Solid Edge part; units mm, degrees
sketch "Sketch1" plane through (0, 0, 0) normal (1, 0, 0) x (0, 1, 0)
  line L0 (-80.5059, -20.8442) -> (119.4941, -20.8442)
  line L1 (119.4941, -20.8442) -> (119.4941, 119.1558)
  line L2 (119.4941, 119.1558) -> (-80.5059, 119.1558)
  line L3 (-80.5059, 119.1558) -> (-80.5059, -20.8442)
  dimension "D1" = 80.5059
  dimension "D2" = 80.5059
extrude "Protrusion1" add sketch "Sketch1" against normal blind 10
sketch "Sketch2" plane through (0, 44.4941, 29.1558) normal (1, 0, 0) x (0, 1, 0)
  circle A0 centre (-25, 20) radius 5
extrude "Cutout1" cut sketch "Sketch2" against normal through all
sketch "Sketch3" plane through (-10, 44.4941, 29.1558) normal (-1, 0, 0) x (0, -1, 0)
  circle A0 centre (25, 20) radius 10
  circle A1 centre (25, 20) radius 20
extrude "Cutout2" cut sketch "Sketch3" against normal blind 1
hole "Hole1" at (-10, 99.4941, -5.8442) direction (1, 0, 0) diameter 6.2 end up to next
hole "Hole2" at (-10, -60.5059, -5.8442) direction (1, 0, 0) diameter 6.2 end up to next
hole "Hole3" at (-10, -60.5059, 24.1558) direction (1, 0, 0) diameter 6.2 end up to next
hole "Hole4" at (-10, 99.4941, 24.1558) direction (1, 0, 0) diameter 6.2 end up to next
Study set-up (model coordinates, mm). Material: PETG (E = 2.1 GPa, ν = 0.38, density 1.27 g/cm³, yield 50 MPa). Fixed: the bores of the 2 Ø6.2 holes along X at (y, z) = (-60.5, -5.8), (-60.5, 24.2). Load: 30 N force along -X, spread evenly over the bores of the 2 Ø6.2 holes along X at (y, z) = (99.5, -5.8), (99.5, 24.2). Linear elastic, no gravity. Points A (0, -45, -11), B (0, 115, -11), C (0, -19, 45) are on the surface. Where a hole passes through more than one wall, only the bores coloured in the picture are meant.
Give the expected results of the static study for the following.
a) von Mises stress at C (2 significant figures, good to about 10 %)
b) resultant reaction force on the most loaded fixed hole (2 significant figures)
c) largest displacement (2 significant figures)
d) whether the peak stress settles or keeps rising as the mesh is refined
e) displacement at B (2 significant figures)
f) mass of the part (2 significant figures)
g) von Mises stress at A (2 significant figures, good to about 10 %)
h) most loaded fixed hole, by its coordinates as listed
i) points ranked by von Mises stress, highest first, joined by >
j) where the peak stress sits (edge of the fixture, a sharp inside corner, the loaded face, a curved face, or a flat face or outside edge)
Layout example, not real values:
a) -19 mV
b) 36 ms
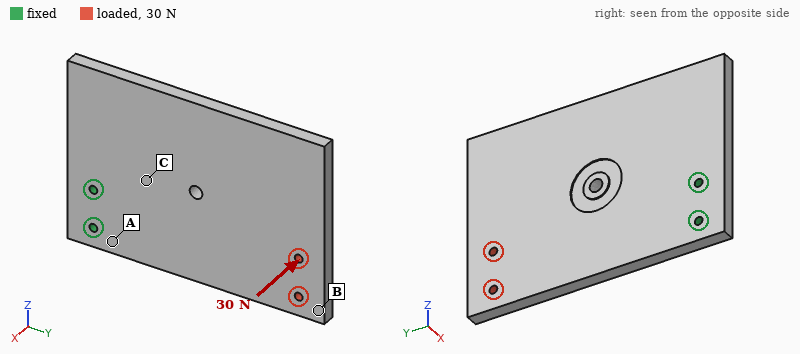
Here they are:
a) 1.5 MPa
b) 17 N
c) 2.9 mm
d) keeps rising
e) 2.8 mm
f) 350 g
g) 2.9 MPa
h) (-60.5, 24.2)
i) A > C > B
j) edge of the fixture
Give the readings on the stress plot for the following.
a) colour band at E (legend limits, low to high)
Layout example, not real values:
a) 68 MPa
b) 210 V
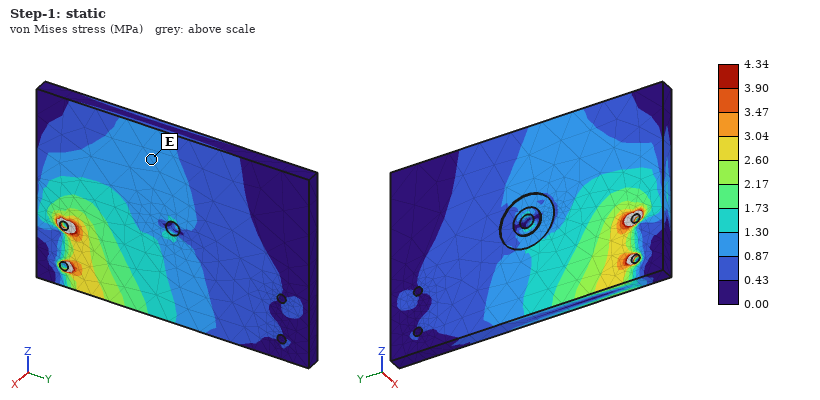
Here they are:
a) 0.87 to 1.30 MPa
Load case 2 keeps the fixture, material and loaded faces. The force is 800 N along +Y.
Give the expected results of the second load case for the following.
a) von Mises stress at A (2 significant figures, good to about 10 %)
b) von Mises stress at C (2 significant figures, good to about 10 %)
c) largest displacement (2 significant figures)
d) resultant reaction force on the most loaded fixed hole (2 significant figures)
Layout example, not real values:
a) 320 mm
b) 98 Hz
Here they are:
a) 1.5 MPa
b) 0.56 MPa
c) 0.14 mm
d) 400 N
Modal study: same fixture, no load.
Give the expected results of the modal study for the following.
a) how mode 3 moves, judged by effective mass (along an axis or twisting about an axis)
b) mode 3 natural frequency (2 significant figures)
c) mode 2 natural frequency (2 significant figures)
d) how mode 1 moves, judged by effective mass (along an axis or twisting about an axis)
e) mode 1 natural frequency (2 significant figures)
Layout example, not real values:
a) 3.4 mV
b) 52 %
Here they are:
a) along Z
b) 230 Hz
c) 130 Hz
d) along X
e) 52 Hz
